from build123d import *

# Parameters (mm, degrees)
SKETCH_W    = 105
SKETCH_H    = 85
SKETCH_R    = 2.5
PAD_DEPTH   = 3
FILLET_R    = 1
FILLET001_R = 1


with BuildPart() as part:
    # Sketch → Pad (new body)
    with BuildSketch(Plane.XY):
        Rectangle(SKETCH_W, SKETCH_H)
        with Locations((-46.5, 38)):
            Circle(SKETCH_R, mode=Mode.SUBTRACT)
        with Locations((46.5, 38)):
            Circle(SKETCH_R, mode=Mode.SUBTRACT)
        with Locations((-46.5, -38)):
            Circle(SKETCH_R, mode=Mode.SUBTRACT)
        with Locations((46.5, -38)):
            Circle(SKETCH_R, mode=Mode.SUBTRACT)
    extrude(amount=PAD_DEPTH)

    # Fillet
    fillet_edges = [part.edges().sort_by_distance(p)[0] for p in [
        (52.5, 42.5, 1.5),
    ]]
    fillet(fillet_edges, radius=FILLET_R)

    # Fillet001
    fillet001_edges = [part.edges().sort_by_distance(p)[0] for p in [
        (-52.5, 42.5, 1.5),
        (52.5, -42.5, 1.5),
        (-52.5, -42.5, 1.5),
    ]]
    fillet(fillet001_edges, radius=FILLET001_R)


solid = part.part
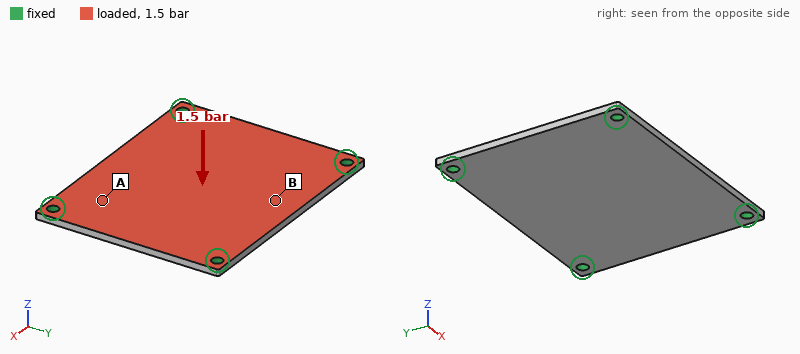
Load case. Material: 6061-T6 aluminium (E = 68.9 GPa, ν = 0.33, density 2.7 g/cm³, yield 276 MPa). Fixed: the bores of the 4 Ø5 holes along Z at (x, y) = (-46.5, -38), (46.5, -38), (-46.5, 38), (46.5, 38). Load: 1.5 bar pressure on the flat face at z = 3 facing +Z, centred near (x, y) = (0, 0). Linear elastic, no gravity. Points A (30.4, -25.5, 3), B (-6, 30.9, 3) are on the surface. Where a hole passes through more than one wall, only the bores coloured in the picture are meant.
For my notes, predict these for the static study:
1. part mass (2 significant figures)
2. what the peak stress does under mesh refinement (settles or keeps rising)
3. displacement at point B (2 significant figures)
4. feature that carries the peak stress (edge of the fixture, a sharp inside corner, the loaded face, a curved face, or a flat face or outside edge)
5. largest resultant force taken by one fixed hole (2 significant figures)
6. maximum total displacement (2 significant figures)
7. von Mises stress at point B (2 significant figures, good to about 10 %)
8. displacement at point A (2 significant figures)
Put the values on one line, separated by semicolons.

72 g; keeps rising; 0.28 mm; edge of the fixture; 330 N; 0.36 mm; 43 MPa; 0.15 mm
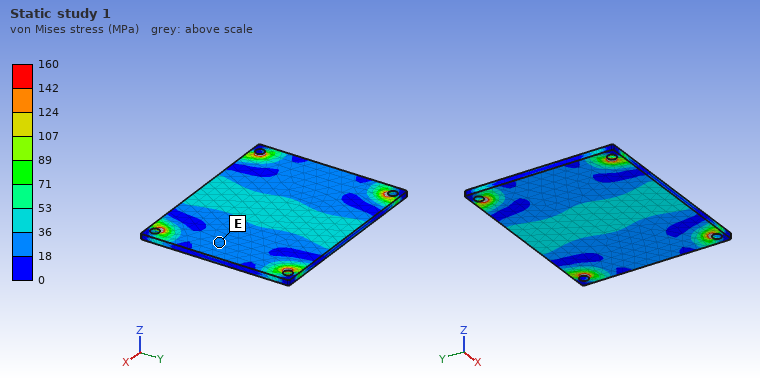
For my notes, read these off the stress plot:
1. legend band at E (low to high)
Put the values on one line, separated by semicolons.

18 to 36 MPa
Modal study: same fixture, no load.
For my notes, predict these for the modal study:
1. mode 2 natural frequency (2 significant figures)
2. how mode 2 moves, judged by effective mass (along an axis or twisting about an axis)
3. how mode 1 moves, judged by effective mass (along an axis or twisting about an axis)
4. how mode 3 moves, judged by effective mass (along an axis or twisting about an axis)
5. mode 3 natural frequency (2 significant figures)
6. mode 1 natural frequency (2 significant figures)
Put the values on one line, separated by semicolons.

2200 Hz; twisting about X; along Z; twisting about Y; 2800 Hz; 1400 Hz
